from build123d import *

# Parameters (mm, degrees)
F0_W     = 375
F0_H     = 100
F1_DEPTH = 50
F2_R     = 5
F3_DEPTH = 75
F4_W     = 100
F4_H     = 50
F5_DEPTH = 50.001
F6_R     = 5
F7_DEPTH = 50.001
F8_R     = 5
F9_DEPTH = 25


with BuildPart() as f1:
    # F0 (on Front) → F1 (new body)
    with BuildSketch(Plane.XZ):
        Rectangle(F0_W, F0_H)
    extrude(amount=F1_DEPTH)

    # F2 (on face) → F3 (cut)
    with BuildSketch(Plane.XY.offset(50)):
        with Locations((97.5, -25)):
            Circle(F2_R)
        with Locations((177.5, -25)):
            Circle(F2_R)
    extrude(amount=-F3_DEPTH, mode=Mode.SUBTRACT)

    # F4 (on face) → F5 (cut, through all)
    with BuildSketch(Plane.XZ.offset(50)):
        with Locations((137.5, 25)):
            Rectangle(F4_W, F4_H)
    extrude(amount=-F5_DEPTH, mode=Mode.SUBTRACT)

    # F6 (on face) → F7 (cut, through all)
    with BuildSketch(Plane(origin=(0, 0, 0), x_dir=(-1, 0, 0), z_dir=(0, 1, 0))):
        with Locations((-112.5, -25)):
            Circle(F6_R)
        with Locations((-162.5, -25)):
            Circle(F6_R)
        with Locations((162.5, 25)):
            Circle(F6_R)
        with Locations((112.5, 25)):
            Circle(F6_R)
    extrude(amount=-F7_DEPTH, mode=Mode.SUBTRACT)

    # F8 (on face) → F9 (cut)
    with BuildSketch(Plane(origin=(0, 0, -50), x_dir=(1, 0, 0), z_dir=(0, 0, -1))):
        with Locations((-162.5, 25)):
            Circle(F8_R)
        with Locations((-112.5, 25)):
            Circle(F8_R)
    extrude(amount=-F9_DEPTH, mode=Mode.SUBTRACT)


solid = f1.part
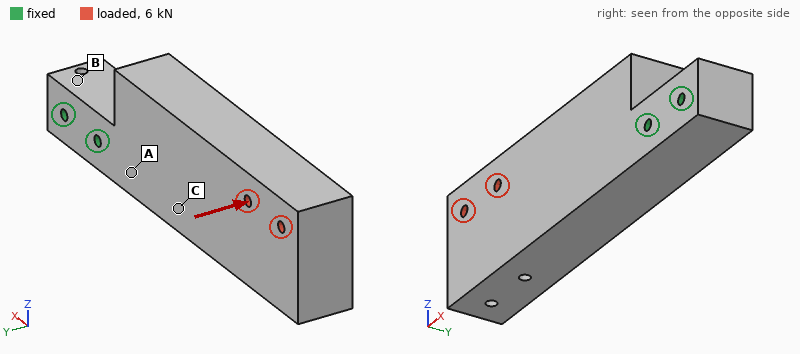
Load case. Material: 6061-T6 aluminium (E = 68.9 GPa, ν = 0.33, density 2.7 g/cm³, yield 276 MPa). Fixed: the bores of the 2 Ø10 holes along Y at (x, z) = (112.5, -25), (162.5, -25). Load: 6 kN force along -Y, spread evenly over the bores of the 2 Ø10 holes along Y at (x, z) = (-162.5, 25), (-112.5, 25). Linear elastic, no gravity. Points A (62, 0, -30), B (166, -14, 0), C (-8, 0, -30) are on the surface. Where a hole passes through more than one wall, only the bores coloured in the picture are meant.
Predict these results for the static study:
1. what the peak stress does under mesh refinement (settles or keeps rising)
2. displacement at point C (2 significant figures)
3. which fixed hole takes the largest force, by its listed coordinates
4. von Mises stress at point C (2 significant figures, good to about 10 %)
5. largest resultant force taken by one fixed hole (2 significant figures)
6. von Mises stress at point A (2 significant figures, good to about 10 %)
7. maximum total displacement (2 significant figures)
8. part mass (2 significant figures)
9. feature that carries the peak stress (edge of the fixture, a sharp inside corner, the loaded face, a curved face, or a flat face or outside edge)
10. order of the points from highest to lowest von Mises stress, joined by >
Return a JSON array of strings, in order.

["keeps rising", "0.26 mm", "(112.5, -25)", "20 MPa", "12 kN", "45 MPa", "0.99 mm", "4.3 kg", "edge of the fixture", "A > C > B"]
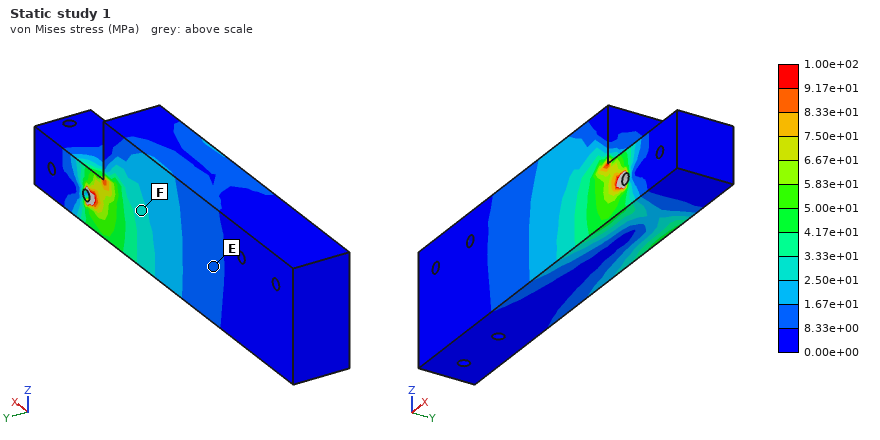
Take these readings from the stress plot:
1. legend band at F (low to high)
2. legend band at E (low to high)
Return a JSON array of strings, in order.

["2.50e+01 to 3.33e+01 MPa", "8.33e+00 to 1.67e+01 MPa"]
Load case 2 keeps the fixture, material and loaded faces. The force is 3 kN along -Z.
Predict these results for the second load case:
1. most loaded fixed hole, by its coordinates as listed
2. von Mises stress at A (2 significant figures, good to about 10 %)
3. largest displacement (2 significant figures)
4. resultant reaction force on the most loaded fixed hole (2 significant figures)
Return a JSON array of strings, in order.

["(112.5, -25)", "11 MPa", "0.47 mm", "14 kN"]
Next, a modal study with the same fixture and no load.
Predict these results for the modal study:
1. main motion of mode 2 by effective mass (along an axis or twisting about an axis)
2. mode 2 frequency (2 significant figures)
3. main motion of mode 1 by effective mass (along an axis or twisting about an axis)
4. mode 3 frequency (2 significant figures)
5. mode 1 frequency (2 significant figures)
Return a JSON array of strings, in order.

["along Y", "340 Hz", "along Z", "1400 Hz", "330 Hz"]
